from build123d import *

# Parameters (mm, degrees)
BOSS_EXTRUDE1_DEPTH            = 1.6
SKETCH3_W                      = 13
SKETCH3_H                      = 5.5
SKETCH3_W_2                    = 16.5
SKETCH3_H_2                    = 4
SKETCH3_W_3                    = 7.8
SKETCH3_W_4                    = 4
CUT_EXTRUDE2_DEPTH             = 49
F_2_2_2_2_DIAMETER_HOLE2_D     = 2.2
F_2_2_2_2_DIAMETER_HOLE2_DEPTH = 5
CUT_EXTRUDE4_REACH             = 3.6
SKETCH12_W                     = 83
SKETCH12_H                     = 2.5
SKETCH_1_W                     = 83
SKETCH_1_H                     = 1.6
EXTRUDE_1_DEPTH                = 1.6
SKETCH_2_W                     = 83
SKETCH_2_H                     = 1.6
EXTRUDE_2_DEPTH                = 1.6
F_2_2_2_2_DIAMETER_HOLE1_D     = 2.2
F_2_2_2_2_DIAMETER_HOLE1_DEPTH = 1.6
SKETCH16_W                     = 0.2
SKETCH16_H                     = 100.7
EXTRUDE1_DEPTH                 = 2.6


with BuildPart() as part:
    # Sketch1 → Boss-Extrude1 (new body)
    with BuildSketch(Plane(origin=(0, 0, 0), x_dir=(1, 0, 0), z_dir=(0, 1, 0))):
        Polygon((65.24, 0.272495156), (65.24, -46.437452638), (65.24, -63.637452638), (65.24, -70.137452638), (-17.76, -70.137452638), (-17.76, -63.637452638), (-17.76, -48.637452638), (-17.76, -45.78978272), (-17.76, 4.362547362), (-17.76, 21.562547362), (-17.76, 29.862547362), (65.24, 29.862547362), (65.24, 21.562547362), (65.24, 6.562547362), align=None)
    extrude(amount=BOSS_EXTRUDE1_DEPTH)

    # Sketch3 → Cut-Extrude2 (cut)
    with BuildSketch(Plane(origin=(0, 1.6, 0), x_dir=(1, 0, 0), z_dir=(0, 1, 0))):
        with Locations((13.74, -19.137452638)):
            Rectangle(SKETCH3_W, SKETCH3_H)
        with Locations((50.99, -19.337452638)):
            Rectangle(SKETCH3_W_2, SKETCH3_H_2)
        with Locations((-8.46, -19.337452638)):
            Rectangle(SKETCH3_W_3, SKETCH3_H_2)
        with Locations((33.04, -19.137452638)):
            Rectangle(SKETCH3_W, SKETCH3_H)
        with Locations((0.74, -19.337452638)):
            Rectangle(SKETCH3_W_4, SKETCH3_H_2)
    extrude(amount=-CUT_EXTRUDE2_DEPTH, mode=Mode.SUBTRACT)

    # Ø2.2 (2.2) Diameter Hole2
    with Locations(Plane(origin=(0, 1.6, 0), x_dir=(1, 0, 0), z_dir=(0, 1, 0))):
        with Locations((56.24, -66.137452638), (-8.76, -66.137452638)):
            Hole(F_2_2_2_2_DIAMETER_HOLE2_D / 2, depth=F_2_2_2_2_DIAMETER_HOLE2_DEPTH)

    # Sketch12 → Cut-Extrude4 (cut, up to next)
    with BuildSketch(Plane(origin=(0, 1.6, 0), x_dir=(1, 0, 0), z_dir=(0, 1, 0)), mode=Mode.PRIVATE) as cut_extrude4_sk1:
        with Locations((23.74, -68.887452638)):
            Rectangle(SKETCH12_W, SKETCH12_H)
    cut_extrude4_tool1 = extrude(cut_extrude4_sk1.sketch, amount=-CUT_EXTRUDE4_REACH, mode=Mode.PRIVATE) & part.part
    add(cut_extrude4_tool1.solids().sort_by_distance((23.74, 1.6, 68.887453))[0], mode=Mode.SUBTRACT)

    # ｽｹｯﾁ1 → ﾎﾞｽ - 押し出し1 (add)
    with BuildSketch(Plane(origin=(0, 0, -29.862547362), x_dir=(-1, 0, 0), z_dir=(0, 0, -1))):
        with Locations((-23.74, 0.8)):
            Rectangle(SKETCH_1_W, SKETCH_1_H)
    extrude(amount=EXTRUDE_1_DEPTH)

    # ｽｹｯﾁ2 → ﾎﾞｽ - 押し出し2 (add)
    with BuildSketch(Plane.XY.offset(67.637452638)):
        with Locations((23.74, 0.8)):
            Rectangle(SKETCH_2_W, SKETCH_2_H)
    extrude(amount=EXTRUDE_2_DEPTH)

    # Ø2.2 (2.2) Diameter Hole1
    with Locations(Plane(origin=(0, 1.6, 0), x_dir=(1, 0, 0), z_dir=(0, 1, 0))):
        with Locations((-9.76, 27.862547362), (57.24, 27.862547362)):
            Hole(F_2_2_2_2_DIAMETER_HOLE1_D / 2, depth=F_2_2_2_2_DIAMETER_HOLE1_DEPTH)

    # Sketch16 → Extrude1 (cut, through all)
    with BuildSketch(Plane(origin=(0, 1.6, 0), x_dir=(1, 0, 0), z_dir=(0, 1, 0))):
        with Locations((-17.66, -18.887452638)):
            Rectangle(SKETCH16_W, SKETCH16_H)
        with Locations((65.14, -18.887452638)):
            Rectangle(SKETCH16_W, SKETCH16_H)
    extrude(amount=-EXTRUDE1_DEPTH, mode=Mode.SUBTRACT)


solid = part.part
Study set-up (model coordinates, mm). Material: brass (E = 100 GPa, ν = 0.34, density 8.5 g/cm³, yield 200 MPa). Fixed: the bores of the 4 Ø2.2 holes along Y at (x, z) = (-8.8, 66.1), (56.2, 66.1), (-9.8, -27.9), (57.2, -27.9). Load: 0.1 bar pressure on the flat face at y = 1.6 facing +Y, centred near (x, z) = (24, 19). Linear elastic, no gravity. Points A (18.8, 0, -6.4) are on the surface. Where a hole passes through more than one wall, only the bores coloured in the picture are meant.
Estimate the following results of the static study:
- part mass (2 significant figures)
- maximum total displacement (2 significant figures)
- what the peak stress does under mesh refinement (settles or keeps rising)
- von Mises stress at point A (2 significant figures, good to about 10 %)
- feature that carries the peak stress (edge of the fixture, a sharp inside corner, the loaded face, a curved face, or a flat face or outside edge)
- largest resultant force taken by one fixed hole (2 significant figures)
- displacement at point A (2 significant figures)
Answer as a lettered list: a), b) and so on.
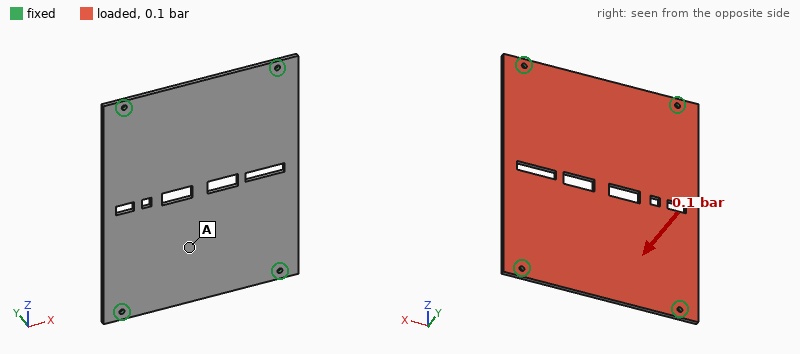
a) 110 g
b) 0.13 mm
c) keeps rising
d) 5.9 MPa
e) edge of the fixture
f) 20 N
g) 0.080 mm
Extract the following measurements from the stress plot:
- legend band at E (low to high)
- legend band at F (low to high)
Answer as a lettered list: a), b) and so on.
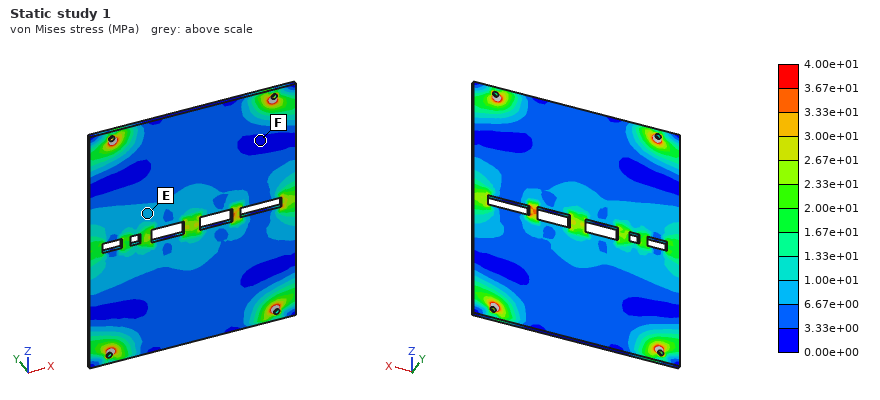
a) 6.67e+00 to 1.00e+01 MPa
b) 0.00e+00 to 3.33e+00 MPa
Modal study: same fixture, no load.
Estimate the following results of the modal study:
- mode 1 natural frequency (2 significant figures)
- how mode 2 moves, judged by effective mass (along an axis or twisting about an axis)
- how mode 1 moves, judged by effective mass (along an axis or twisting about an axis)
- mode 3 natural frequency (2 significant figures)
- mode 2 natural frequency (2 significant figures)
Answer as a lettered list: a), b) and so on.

a) 460 Hz
b) twisting about Z
c) along Y
d) 1100 Hz
e) 760 Hz
